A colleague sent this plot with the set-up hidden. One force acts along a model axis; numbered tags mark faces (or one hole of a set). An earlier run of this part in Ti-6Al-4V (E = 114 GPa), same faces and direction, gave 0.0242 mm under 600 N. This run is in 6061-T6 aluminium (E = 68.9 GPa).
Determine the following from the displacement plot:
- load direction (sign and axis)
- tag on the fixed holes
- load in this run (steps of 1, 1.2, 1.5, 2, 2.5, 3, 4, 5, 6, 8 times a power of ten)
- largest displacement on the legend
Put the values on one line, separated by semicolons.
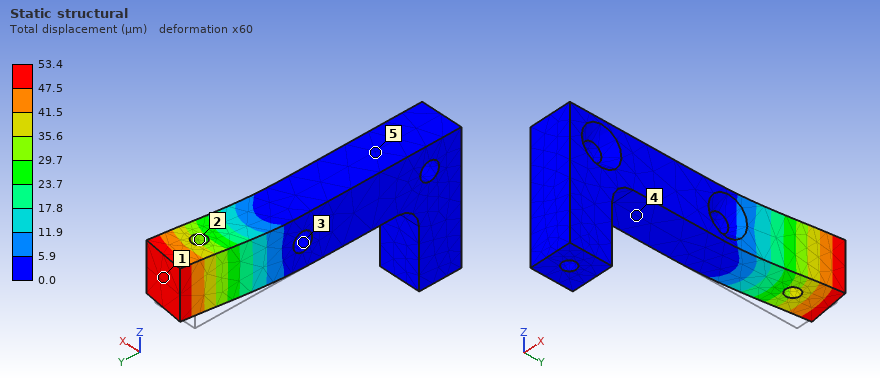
+X; 3; 800 N; 53.4 µm
